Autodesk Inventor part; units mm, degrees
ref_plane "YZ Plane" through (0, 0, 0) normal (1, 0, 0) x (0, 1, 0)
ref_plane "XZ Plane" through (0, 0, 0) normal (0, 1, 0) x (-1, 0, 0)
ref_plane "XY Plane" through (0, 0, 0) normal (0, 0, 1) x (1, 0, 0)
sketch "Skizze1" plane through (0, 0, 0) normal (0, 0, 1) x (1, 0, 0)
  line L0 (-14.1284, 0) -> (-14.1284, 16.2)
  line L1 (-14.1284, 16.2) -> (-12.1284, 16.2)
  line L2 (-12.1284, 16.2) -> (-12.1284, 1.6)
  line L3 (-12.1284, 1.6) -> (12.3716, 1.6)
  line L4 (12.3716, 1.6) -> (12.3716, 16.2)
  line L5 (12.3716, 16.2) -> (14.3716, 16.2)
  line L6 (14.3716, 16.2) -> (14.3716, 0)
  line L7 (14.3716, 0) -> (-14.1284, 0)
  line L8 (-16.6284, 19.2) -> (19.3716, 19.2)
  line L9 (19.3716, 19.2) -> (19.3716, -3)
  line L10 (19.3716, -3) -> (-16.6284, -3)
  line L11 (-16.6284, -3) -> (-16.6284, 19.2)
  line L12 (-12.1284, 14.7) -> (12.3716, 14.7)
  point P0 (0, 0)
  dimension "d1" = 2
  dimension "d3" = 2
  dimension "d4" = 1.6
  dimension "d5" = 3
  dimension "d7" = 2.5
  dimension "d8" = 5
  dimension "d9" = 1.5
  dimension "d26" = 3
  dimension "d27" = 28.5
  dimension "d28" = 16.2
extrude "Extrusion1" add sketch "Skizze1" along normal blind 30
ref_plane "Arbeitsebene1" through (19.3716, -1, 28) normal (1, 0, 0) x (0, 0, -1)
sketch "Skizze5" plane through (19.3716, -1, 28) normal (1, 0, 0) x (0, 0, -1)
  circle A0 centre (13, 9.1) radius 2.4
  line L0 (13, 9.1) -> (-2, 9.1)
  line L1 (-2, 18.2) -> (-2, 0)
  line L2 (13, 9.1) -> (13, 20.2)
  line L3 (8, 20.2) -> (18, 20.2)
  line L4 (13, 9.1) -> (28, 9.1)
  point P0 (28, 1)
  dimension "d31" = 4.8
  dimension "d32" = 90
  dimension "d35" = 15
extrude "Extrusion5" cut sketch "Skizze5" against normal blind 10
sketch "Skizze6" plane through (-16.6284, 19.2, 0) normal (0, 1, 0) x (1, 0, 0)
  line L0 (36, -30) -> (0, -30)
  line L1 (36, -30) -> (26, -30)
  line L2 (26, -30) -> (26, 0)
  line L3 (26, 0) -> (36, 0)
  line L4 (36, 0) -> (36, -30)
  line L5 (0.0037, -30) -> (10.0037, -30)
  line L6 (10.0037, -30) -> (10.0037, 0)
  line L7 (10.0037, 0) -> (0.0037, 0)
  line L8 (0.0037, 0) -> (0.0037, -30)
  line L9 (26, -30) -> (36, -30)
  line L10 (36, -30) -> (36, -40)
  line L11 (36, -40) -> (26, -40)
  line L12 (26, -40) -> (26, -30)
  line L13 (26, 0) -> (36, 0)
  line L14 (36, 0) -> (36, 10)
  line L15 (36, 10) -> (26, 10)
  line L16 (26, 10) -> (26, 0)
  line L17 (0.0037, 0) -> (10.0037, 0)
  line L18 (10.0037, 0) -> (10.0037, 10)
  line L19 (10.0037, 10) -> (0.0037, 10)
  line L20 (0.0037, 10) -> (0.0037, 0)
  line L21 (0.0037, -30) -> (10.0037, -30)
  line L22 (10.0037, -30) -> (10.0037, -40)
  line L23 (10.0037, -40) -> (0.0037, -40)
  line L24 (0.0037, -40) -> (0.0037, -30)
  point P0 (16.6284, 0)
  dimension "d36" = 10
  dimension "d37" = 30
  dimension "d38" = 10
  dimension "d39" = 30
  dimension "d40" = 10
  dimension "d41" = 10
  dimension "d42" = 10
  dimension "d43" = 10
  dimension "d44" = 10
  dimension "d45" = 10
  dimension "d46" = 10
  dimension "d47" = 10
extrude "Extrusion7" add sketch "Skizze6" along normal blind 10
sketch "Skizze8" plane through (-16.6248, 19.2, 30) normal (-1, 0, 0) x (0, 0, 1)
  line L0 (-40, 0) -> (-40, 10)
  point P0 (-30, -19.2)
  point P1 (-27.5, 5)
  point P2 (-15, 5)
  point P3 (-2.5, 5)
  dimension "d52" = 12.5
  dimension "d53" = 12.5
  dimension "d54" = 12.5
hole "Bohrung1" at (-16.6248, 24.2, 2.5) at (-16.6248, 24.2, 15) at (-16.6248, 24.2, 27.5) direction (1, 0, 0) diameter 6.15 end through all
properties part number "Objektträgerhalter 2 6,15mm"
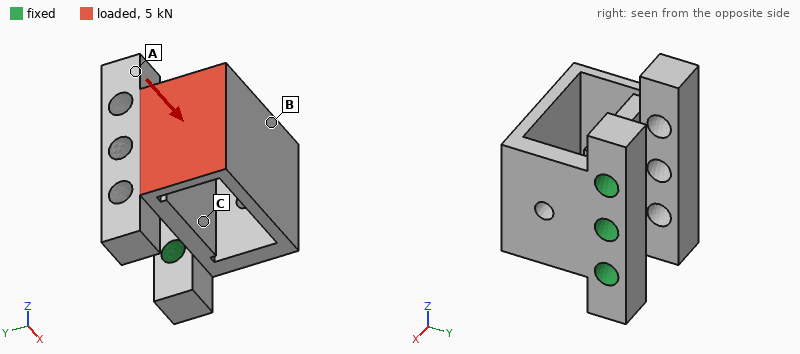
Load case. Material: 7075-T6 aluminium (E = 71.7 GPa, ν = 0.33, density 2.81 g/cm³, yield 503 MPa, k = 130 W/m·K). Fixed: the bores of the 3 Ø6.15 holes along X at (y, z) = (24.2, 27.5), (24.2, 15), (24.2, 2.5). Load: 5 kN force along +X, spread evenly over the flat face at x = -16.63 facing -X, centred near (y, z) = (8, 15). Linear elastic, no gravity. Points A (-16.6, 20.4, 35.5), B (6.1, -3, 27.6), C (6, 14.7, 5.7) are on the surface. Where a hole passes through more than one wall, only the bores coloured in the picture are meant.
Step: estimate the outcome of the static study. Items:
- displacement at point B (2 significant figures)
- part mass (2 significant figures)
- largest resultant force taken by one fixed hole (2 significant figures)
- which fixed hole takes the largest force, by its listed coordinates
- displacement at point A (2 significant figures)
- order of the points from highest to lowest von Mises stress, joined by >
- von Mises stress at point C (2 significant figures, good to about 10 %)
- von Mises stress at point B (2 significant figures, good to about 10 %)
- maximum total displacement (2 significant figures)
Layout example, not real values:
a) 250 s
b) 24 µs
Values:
a) 0.29 mm
b) 54 g
c) 2.0 kN
d) (24.2, 15)
e) 0.25 mm
f) C > B > A
g) 100 MPa
h) 43 MPa
i) 0.34 mm
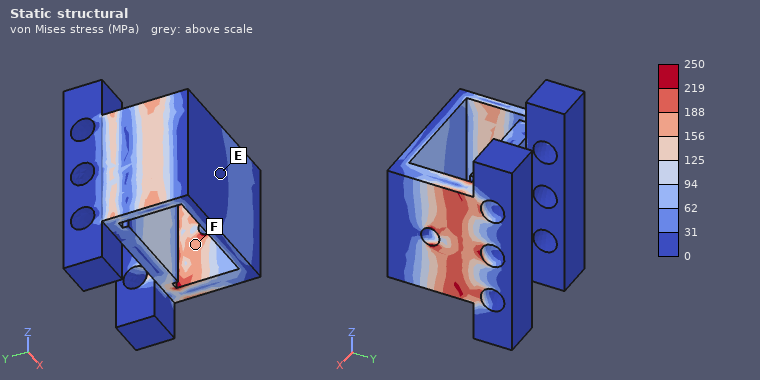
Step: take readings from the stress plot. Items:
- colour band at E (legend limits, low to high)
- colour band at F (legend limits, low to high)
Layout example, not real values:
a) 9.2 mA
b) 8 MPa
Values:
a) 0 to 31 MPa
b) 156 to 188 MPa
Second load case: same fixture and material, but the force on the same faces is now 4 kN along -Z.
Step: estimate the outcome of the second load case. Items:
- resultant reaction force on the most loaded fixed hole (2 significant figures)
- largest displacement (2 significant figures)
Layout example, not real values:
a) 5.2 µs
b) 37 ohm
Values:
a) 5.1 kN
b) 0.35 mm
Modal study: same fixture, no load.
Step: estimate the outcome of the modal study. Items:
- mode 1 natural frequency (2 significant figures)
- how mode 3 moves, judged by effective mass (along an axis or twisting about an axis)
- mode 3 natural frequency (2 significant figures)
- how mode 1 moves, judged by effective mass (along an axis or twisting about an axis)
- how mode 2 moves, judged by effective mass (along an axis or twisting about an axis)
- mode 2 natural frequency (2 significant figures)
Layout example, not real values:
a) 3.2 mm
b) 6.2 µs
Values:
a) 2200 Hz
b) along X
c) 5900 Hz
d) along Y
e) twisting about X
f) 4000 Hz
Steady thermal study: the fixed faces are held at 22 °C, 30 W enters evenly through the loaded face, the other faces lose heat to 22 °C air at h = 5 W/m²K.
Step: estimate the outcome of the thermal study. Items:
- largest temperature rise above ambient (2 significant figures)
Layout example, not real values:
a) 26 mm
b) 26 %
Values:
a) 41 K
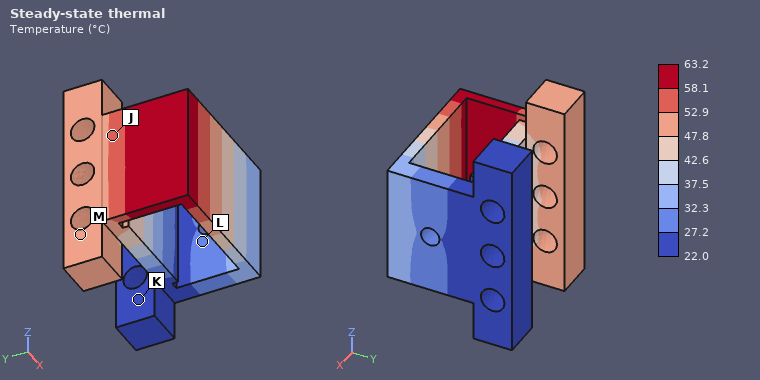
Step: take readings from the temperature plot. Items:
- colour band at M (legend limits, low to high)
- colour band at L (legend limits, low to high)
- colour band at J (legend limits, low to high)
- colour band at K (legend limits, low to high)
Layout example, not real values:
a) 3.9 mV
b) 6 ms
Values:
a) 47.8 to 52.9 °C
b) 27.2 to 32.3 °C
c) 52.9 to 58.1 °C
d) 22.0 to 27.2 °C
